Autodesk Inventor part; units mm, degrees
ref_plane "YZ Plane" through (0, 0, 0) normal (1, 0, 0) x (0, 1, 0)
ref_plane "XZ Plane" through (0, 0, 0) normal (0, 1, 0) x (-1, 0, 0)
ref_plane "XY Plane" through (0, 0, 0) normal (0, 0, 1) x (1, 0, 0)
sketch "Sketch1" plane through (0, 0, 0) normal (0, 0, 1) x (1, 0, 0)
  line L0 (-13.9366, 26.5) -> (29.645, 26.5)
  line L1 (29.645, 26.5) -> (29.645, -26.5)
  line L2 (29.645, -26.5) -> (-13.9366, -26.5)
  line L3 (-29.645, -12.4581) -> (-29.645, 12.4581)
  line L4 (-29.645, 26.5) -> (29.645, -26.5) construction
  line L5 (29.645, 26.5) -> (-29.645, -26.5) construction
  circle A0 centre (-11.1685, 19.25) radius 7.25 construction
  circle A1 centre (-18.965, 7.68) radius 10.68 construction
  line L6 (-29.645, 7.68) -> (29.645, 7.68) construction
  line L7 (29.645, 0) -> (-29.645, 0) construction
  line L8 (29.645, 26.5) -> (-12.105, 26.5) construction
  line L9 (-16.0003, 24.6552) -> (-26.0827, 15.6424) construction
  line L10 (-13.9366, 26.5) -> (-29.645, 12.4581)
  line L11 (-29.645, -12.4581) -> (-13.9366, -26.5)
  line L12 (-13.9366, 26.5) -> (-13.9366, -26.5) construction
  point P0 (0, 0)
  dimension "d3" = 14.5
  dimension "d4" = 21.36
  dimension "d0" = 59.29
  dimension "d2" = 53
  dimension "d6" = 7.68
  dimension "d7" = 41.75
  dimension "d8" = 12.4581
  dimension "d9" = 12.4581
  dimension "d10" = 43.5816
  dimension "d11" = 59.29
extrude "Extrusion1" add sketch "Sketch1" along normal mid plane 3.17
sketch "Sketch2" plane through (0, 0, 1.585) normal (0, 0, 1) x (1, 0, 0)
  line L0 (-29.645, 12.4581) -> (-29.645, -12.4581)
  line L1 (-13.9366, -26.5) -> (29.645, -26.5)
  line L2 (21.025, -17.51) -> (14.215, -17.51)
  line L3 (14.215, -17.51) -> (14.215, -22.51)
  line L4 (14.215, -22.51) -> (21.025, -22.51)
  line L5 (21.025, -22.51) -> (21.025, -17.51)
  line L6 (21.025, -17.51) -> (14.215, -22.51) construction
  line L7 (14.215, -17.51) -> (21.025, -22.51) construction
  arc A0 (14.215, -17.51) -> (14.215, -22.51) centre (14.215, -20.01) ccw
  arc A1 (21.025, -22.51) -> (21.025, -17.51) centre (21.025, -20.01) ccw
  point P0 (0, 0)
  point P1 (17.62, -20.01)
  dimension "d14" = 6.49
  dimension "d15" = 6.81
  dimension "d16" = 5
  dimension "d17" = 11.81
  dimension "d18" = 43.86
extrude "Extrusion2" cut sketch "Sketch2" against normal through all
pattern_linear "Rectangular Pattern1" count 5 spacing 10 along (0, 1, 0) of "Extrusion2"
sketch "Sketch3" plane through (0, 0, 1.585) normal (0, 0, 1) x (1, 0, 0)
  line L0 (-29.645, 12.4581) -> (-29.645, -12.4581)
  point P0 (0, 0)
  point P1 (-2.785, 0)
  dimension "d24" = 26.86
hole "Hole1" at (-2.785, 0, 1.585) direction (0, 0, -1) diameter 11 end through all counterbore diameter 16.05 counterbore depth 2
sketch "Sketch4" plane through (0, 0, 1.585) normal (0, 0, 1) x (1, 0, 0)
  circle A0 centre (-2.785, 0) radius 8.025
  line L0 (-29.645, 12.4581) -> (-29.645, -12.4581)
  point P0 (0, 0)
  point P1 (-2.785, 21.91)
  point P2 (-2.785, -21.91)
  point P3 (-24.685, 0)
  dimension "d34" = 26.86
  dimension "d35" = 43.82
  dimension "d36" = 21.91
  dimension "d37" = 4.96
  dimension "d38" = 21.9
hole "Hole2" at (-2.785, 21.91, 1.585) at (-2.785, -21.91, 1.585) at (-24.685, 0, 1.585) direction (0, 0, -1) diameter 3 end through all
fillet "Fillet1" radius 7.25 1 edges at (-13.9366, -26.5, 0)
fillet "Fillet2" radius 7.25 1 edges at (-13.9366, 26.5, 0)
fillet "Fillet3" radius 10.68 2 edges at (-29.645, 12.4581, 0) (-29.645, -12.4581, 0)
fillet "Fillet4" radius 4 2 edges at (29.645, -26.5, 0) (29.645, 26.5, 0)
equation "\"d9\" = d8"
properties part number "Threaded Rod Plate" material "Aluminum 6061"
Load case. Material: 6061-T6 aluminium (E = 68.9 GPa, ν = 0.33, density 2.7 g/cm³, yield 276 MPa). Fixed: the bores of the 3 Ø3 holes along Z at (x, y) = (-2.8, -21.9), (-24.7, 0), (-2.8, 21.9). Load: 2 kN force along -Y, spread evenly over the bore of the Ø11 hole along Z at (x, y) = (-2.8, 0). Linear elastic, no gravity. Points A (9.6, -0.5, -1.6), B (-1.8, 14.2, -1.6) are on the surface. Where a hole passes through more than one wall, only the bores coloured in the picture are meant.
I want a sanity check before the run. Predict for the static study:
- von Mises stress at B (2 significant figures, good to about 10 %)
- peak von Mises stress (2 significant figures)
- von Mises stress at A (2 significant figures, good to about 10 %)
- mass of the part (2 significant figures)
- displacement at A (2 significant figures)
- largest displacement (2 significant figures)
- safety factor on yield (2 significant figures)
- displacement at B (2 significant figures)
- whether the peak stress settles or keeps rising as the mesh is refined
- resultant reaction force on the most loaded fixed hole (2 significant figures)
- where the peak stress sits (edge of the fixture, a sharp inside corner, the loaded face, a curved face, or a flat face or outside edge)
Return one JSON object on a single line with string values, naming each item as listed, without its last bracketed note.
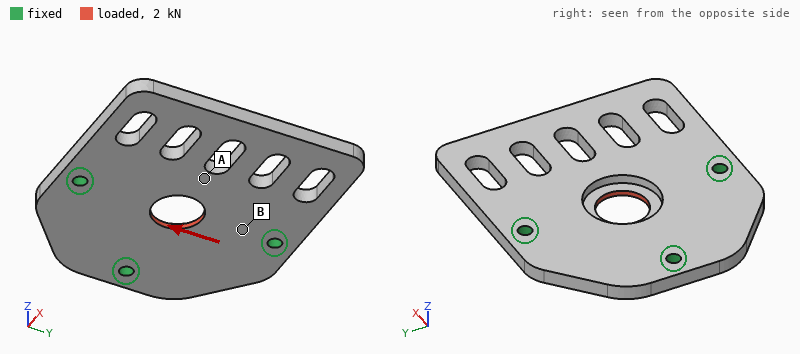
{"von Mises stress at B": "32 MPa", "peak von Mises stress": "89 MPa", "von Mises stress at A": "12 MPa", "mass of the part": "21 g", "displacement at A": "4.7 µm", "largest displacement": "10 µm", "safety factor on yield": "3.1", "displacement at B": "2.9 µm", "whether the peak stress settles or keeps rising as the mesh is refined": "settles", "resultant reaction force on the most loaded fixed hole": "830 N", "where the peak stress sits": "the loaded face"}
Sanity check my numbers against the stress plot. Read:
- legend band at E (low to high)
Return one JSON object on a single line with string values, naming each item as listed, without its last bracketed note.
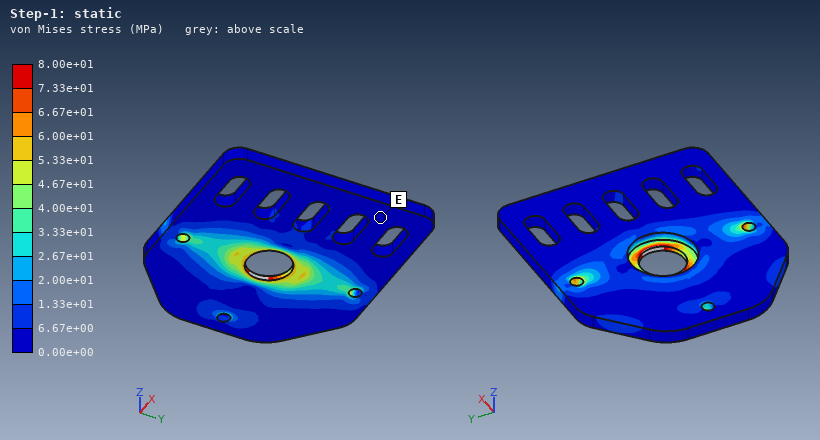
{"legend band at E": "0.00e+00 to 6.67e+00 MPa"}
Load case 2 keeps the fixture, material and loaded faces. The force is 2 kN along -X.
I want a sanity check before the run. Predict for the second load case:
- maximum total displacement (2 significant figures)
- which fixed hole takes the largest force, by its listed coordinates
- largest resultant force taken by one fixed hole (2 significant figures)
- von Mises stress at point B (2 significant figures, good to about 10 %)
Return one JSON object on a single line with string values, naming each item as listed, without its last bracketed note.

{"maximum total displacement": "43 µm", "which fixed hole takes the largest force, by its listed coordinates": "(-24.7, 0)", "largest resultant force taken by one fixed hole": "800 N", "von Mises stress at point B": "14 MPa"}
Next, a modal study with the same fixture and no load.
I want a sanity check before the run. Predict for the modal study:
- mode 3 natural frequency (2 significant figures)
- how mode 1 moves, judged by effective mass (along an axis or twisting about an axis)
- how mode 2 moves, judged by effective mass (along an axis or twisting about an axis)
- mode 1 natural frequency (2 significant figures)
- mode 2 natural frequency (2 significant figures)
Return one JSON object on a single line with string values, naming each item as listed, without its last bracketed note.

{"mode 3 natural frequency": "7300 Hz", "how mode 1 moves, judged by effective mass": "along Z", "how mode 2 moves, judged by effective mass": "twisting about X", "mode 1 natural frequency": "2100 Hz", "mode 2 natural frequency": "4100 Hz"}
